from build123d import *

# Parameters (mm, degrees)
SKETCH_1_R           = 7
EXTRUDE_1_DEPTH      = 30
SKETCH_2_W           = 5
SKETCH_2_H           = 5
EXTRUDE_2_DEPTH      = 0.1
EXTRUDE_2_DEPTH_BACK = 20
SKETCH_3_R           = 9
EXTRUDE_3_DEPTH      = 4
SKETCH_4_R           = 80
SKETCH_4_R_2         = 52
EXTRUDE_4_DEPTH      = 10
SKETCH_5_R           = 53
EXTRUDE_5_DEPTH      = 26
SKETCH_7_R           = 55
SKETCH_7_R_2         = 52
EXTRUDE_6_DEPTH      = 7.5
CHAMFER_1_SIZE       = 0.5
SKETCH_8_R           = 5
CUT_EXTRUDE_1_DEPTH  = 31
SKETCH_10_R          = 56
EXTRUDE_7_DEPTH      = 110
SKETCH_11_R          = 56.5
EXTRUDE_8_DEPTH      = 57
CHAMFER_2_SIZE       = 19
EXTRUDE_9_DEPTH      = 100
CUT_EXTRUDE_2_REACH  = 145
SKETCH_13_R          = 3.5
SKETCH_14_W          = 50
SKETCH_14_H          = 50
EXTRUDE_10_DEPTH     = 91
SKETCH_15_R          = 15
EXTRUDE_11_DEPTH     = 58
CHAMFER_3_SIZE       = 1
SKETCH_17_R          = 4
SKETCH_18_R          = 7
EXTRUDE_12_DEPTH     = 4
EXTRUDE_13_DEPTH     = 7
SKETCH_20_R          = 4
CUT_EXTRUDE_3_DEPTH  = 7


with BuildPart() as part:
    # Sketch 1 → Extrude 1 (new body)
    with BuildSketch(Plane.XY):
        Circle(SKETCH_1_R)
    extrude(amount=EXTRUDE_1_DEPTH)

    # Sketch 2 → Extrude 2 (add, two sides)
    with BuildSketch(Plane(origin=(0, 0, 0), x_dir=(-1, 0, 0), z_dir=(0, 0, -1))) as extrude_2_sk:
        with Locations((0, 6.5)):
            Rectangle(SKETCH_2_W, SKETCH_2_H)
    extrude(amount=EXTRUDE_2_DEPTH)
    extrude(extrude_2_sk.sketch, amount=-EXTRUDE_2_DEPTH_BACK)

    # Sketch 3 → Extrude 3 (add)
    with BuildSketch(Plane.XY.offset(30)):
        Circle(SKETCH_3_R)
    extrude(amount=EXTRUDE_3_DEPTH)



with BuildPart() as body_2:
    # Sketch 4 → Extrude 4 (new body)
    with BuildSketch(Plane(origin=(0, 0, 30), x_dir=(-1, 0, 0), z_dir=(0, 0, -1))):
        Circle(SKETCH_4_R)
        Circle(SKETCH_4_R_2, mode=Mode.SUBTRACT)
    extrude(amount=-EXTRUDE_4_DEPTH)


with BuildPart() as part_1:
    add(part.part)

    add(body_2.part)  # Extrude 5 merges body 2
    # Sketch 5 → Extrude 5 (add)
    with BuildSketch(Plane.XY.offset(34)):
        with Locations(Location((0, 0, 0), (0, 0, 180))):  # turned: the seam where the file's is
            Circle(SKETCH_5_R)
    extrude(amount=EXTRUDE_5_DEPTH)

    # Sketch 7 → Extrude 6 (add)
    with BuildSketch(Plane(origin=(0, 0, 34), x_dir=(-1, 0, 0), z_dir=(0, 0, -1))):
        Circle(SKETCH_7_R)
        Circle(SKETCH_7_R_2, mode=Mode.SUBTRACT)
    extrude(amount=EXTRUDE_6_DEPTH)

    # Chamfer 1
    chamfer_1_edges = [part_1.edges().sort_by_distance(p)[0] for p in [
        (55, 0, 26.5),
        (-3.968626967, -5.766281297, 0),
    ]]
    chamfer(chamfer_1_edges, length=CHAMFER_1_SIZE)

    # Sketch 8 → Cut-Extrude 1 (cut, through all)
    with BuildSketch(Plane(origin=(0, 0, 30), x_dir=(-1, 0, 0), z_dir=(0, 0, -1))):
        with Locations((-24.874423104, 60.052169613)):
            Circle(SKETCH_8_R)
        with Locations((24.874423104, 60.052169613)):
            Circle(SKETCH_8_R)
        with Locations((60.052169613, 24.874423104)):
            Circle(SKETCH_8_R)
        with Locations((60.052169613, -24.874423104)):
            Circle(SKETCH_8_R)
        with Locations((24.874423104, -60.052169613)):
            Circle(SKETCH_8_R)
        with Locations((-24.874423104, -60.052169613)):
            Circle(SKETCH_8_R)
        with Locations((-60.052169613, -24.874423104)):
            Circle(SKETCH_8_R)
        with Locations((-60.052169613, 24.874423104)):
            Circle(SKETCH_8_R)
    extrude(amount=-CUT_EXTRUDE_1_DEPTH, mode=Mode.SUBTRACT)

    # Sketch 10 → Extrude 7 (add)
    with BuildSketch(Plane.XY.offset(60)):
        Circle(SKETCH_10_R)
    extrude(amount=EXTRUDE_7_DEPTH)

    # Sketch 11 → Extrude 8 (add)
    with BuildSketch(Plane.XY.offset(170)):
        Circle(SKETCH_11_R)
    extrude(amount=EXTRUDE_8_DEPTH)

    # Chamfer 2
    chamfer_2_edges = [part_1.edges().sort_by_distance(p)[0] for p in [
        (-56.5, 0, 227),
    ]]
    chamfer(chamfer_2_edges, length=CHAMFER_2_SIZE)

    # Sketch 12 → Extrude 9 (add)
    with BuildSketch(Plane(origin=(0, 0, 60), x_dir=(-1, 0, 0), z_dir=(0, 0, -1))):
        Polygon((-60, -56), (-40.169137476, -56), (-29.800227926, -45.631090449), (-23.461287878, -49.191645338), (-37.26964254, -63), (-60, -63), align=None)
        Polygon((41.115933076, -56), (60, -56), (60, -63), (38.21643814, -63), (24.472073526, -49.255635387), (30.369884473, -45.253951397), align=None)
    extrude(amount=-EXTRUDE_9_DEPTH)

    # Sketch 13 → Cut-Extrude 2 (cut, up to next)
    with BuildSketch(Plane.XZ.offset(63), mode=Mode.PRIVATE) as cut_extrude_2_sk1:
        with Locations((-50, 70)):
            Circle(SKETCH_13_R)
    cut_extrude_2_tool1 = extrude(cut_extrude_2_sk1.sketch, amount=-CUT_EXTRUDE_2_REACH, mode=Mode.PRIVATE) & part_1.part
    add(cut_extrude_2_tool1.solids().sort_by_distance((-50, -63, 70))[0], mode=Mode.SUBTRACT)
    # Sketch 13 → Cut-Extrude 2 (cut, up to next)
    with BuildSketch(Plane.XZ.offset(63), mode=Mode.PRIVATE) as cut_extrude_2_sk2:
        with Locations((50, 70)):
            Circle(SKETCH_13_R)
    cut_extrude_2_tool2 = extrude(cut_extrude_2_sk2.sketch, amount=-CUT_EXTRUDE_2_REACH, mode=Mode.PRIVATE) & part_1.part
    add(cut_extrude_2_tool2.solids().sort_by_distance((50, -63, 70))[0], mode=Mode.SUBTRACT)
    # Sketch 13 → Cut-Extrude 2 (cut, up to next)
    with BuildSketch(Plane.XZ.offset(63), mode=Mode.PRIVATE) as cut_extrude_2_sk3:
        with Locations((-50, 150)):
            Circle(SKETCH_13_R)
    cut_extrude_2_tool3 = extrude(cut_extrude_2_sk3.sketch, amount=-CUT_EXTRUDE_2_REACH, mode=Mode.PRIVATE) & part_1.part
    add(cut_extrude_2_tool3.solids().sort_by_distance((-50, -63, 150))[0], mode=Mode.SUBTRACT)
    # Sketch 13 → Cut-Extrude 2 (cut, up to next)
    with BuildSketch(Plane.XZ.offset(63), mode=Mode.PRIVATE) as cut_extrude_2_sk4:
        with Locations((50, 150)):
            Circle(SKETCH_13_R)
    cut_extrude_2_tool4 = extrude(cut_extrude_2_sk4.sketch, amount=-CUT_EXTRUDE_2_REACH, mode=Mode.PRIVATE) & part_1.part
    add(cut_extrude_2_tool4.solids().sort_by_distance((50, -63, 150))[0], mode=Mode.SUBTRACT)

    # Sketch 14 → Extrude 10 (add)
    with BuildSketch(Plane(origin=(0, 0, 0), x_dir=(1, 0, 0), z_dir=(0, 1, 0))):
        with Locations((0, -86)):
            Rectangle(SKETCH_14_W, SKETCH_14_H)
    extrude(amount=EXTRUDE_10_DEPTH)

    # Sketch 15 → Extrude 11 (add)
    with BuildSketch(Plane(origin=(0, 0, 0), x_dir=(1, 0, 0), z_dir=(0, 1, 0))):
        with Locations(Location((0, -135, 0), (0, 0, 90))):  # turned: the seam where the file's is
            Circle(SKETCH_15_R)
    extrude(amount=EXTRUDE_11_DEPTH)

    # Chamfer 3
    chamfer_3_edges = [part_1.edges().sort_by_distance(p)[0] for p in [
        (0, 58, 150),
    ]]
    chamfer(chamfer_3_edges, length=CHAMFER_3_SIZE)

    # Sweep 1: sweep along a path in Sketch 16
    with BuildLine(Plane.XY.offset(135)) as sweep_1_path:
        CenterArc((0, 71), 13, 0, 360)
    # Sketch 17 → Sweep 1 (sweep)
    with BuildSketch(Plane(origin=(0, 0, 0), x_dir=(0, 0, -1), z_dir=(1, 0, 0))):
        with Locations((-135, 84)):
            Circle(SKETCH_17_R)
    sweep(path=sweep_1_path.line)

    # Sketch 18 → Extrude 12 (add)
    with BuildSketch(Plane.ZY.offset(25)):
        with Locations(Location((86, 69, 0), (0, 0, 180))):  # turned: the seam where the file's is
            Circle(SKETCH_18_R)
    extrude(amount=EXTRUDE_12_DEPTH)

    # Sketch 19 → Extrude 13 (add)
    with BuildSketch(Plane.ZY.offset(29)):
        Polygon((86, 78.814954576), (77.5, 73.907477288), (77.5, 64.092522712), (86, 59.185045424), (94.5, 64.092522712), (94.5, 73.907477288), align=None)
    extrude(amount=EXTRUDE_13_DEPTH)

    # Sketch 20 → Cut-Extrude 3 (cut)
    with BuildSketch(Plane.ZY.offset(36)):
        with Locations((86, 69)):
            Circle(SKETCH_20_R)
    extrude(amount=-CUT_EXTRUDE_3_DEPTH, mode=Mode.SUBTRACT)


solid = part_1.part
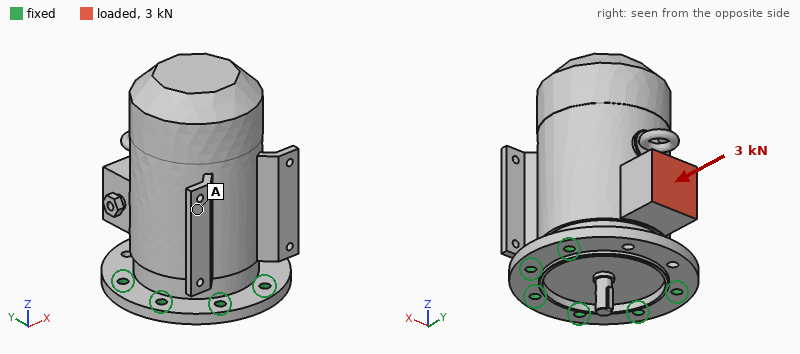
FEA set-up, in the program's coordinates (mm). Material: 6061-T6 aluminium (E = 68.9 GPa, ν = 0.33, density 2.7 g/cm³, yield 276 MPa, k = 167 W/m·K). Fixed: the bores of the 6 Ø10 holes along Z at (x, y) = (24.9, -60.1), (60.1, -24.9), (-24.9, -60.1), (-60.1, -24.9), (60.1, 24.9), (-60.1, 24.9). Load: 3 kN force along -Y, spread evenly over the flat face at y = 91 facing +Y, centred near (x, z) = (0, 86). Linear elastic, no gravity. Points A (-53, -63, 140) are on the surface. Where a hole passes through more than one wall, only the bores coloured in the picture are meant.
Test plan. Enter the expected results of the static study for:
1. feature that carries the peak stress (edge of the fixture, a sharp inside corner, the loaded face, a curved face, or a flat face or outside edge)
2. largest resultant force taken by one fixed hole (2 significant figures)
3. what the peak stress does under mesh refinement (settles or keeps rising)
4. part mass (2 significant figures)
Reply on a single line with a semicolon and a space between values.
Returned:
edge of the fixture; 1.2 kN; keeps rising; 5.7 kg
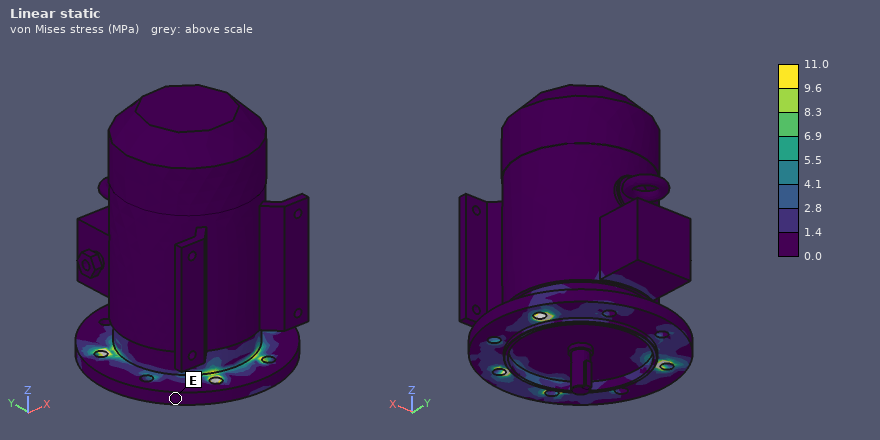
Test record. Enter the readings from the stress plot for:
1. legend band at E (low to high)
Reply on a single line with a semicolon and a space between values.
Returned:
0.0 to 1.4 MPa
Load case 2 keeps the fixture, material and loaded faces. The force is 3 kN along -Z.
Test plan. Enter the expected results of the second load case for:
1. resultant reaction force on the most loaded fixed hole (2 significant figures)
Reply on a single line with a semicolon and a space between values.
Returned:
3.1 kN
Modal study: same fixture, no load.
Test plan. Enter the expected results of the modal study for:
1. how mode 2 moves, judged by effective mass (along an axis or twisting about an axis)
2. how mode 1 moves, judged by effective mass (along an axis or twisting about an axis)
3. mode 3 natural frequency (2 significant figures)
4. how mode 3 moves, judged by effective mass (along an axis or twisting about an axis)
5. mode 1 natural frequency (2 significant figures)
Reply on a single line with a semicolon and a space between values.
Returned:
along X; along Y; 2500 Hz; along Z; 680 Hz
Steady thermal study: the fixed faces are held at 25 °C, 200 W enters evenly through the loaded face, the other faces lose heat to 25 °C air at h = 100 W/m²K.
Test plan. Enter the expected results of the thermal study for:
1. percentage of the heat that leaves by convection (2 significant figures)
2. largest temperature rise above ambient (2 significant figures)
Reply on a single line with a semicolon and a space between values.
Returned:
52 %; 34 K
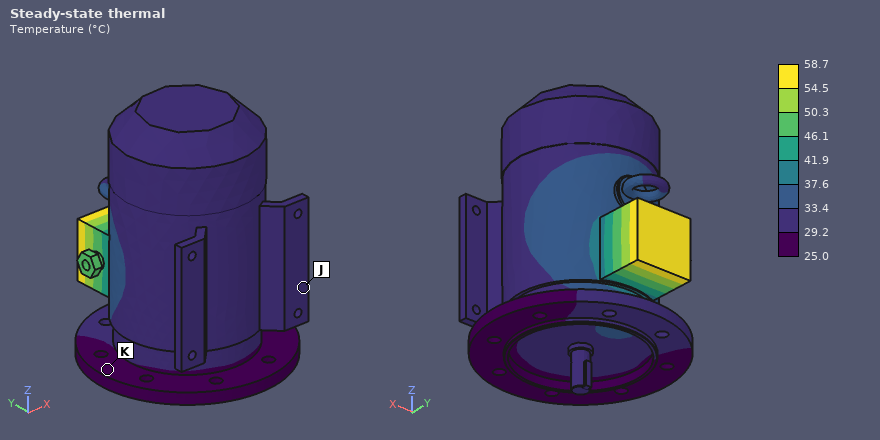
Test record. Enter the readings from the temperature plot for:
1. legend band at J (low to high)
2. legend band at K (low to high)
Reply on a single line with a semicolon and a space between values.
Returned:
29.2 to 33.4 °C; 25.0 to 29.2 °C
